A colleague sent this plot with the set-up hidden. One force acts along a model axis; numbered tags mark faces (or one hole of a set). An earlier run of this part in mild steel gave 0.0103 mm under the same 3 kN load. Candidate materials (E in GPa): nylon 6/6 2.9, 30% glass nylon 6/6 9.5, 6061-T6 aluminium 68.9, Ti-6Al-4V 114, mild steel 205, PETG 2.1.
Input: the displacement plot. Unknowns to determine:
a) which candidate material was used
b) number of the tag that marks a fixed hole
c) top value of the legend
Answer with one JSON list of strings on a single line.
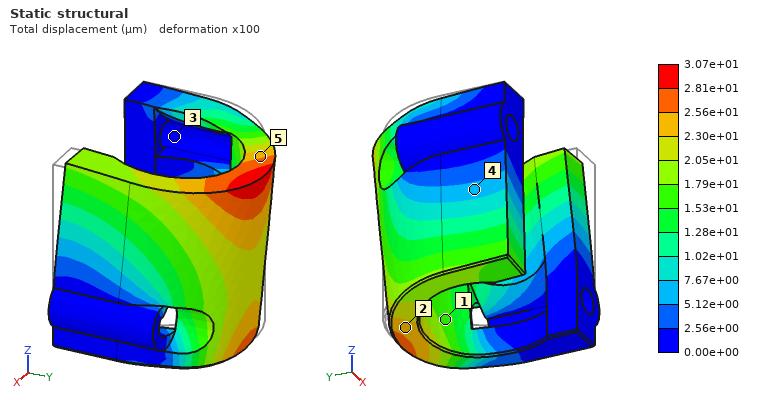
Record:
["6061-T6 aluminium", "3", "3.07e+01 µm"]
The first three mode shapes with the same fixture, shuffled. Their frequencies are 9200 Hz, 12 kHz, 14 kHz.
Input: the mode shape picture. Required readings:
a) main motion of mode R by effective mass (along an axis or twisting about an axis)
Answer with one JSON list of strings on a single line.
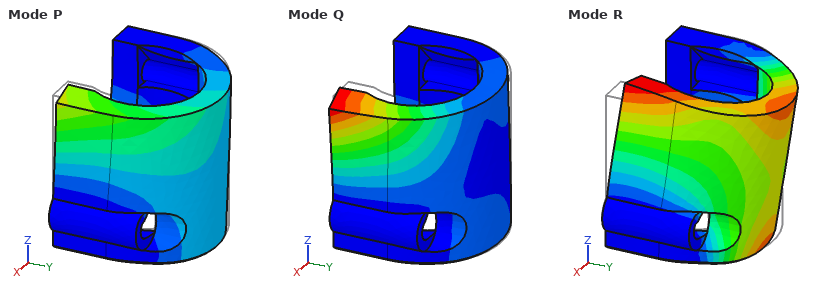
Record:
["along X"]
